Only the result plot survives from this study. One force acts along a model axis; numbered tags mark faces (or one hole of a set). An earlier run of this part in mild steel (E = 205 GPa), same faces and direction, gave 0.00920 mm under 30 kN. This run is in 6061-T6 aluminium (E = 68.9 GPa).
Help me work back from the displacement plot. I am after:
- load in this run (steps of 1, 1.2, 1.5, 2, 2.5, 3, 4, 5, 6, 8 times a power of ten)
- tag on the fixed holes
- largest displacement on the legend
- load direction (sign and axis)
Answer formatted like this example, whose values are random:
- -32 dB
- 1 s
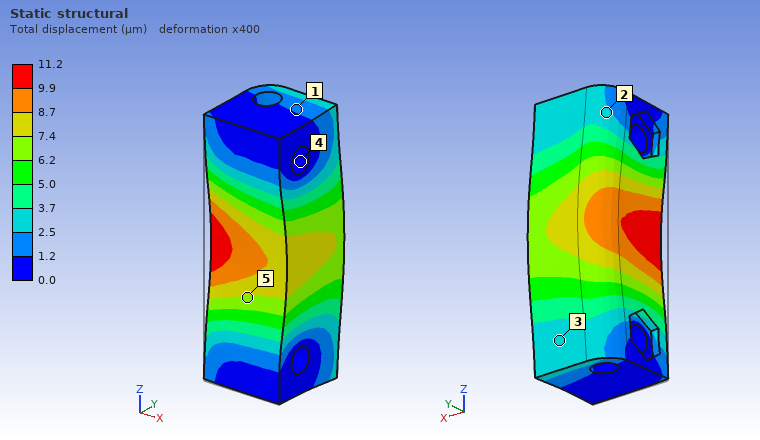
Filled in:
- 12 kN
- 4
- 11.2 µm
- +Y
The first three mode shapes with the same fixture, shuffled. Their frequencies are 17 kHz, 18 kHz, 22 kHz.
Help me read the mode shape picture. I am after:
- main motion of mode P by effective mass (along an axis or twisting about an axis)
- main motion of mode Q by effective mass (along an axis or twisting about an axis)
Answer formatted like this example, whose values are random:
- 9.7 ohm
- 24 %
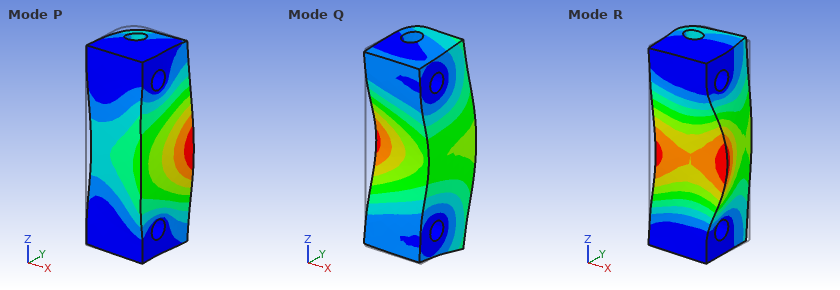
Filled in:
- along X
- along Y
